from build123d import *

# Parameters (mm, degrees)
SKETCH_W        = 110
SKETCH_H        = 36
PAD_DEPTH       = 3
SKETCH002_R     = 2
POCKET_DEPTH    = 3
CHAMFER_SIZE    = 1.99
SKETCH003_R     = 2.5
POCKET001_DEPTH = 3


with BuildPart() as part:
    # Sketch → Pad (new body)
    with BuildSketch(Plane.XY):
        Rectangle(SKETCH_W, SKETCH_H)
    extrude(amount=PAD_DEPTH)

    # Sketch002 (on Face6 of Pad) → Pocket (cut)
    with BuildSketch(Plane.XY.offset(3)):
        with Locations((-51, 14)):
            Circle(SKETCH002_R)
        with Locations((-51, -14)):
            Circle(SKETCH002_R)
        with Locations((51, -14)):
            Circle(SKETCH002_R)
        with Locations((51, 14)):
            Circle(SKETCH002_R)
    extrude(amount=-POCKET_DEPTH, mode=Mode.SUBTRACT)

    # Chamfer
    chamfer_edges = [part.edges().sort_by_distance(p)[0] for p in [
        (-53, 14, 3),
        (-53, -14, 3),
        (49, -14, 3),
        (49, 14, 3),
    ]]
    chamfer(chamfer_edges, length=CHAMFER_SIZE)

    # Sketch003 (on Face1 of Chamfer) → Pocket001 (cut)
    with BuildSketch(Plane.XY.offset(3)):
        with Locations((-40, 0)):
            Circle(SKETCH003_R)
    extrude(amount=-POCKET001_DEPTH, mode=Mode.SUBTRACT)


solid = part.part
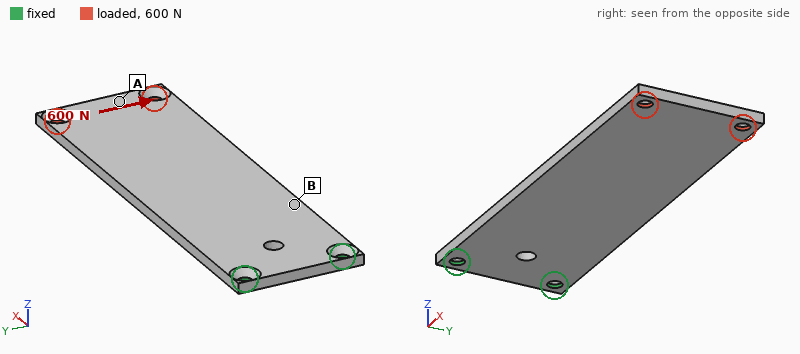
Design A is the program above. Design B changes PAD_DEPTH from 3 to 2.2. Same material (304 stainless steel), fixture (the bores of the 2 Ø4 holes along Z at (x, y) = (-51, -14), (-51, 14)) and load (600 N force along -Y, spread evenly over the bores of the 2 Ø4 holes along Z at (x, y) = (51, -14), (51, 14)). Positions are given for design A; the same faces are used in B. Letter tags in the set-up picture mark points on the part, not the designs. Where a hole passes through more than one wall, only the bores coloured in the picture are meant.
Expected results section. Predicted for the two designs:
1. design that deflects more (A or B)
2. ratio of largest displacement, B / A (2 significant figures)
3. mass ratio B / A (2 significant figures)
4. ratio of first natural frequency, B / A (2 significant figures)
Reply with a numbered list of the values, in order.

1. B
2. 2.0
3. 0.73
4. 0.67
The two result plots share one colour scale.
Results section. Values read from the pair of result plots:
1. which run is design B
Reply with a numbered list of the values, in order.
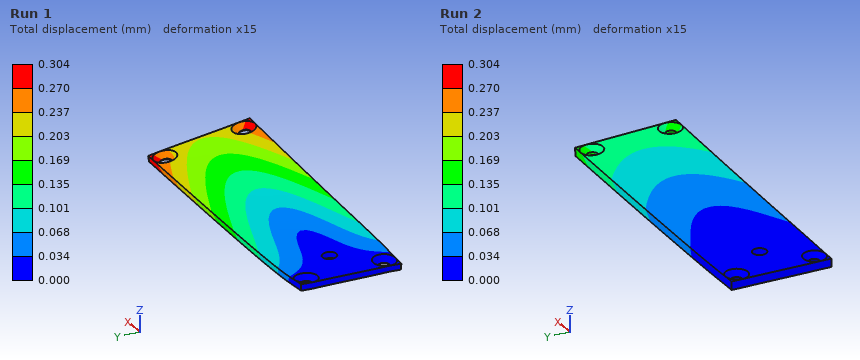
1. Run 1
